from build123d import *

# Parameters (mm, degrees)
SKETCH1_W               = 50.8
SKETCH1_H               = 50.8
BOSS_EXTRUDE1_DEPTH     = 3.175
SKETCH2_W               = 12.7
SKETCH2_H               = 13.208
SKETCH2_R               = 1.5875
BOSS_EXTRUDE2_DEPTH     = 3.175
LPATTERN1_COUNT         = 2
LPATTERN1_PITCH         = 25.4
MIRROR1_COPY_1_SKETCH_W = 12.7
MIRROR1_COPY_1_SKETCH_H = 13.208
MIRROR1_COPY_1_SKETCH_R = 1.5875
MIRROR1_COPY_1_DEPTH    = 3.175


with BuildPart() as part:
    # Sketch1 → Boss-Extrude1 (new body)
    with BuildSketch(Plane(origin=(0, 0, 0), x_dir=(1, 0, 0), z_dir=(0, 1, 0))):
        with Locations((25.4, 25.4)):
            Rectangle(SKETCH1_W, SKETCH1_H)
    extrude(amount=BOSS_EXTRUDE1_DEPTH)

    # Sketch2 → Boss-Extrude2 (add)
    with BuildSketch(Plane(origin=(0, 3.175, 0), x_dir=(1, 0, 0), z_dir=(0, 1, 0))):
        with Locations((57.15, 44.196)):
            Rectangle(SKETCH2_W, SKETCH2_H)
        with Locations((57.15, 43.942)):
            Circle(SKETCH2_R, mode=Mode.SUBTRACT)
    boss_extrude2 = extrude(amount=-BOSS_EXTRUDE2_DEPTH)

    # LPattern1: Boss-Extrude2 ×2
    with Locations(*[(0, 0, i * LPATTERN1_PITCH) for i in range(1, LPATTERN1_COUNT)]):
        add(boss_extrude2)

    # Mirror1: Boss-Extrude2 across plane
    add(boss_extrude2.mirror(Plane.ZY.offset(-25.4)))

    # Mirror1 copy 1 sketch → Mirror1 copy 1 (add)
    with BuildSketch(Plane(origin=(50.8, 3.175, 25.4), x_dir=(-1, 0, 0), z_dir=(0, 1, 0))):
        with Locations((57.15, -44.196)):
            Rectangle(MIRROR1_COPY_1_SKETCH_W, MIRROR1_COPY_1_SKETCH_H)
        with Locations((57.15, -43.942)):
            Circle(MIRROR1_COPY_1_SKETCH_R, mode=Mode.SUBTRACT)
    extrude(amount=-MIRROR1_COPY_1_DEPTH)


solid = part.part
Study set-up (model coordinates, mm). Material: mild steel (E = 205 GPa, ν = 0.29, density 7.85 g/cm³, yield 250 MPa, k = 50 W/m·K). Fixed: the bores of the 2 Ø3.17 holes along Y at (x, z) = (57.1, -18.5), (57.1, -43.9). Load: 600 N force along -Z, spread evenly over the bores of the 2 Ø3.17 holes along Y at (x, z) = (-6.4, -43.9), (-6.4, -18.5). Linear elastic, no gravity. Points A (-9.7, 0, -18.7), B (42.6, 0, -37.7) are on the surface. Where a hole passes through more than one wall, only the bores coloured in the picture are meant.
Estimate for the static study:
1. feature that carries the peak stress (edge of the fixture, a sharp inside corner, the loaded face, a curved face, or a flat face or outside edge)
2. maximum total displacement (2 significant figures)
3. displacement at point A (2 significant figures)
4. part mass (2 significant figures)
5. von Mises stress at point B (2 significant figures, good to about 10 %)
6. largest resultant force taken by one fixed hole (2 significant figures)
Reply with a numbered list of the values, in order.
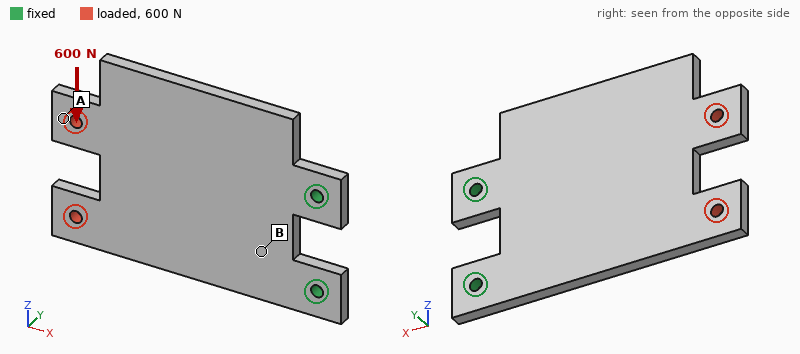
1. edge of the fixture
2. 29 µm
3. 24 µm
4. 80 g
5. 25 MPa
6. 1.4 kN
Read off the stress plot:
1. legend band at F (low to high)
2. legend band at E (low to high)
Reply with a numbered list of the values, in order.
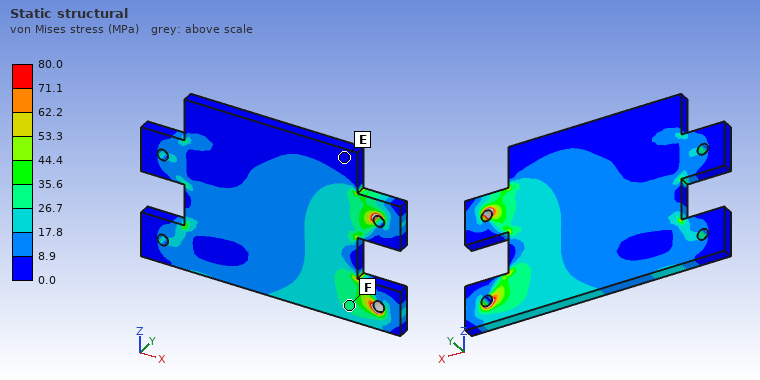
1. 26.7 to 35.6 MPa
2. 0.0 to 8.9 MPa
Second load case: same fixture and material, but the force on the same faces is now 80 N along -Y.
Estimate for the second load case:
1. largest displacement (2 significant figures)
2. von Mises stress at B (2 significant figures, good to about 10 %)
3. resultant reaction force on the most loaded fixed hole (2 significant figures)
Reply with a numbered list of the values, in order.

1. 0.39 mm
2. 47 MPa
3. 41 N
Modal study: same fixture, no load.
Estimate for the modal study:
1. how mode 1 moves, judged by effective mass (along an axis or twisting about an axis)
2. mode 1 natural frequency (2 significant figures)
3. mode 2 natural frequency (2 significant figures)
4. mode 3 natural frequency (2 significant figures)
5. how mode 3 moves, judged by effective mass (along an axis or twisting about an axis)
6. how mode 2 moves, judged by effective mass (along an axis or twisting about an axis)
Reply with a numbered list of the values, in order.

1. along Y
2. 530 Hz
3. 1600 Hz
4. 3400 Hz
5. along Y
6. twisting about X
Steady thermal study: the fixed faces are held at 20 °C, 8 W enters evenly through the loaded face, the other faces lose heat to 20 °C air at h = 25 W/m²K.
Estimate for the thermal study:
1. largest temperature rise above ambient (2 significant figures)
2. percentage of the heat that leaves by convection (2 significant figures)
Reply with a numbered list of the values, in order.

1. 61 K
2. 53 %
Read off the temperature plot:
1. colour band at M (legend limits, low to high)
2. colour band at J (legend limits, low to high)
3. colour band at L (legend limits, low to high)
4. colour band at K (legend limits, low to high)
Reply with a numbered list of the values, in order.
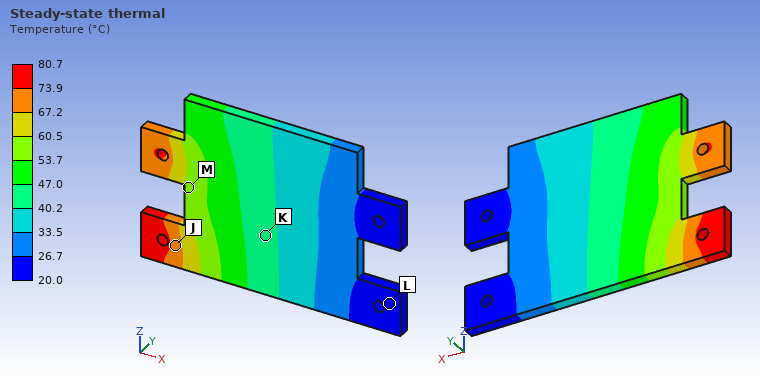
1. 53.7 to 60.5 °C
2. 67.2 to 73.9 °C
3. 20.0 to 26.7 °C
4. 40.2 to 47.0 °C
